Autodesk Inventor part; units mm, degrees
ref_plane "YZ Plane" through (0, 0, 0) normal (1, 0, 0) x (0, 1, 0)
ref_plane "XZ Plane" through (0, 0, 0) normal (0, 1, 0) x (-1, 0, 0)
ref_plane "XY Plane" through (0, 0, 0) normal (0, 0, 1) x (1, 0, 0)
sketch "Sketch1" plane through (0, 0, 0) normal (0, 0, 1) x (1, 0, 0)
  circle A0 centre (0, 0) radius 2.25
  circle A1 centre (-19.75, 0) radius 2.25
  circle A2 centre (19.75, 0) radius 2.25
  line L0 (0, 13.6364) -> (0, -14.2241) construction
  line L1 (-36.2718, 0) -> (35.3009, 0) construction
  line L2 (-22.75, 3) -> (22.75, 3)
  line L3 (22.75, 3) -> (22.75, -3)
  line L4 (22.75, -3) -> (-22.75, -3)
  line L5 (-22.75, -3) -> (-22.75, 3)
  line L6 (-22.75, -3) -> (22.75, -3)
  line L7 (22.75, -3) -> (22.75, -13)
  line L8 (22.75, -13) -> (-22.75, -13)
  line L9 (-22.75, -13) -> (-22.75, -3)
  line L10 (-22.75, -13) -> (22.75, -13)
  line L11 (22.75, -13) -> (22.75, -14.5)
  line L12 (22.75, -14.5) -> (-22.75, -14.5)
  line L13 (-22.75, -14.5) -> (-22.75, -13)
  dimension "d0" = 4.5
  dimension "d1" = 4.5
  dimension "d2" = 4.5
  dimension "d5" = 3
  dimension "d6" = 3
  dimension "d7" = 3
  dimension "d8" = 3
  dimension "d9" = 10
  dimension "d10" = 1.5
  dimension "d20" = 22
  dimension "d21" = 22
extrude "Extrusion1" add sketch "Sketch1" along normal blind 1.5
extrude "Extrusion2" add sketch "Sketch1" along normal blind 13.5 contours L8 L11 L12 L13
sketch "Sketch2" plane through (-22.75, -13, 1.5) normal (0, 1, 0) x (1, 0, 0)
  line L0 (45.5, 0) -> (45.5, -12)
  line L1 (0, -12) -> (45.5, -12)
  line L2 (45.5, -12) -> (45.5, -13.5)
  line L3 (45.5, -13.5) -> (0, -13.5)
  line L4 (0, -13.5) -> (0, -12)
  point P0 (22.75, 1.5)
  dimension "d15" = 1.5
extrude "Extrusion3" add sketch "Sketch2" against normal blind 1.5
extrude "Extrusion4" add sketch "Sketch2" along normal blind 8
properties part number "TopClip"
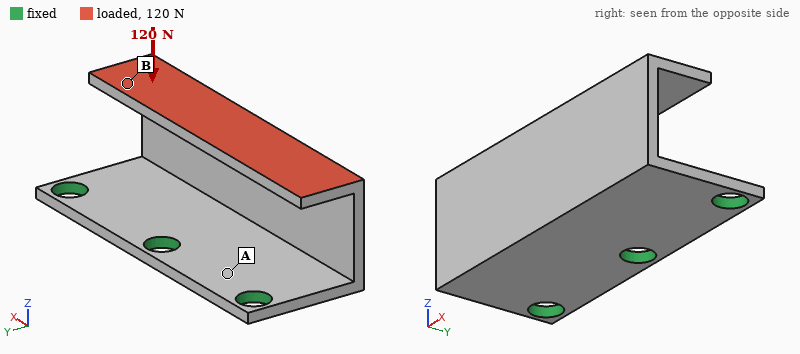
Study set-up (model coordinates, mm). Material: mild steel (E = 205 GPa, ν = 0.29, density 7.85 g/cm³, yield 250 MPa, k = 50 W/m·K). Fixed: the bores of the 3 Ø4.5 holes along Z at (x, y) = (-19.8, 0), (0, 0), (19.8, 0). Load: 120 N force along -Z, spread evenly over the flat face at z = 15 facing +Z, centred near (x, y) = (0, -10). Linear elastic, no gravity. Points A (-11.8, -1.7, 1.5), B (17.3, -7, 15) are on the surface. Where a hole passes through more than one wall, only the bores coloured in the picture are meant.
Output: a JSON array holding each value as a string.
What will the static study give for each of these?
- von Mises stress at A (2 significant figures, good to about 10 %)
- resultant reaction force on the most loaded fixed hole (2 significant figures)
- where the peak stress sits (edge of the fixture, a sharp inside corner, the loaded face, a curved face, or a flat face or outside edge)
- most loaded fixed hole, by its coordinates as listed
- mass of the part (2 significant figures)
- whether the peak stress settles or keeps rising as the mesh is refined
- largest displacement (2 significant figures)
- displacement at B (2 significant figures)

["20 MPa", "52 N", "edge of the fixture", "(0, 0)", "20 g", "keeps rising", "28 µm", "25 µm"]
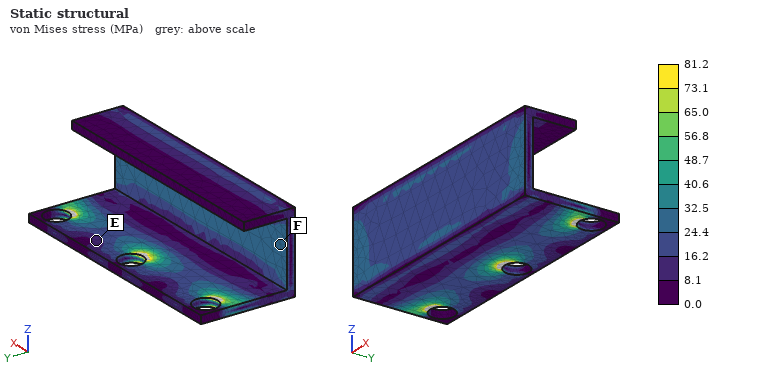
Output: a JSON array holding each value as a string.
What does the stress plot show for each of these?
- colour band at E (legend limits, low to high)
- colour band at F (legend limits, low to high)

["8.1 to 16.2 MPa", "24.4 to 32.5 MPa"]
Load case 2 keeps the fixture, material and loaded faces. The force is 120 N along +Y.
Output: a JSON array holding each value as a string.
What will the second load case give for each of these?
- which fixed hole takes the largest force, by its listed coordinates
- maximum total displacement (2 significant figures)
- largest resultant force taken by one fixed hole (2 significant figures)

["(0, 0)", "0.16 mm", "62 N"]
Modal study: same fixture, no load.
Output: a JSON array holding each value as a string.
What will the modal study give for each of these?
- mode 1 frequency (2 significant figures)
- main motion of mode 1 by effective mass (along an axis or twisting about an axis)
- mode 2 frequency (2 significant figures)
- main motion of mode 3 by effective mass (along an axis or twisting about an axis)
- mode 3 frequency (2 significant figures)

["1600 Hz", "along Y", "2700 Hz", "along Z", "3900 Hz"]
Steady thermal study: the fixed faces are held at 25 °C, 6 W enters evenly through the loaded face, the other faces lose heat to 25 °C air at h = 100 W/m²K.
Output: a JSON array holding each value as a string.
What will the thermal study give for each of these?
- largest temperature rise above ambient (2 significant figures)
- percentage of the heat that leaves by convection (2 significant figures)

["28 K", "65 %"]
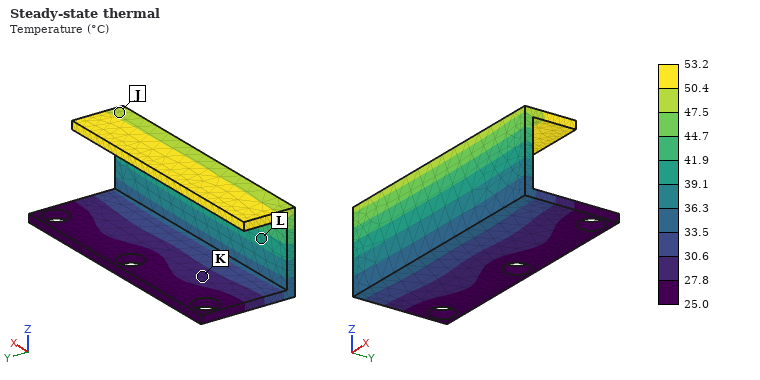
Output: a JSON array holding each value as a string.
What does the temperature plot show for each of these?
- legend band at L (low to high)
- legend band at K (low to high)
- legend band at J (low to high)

["39.1 to 41.9 °C", "27.8 to 30.6 °C", "47.5 to 50.4 °C"]
